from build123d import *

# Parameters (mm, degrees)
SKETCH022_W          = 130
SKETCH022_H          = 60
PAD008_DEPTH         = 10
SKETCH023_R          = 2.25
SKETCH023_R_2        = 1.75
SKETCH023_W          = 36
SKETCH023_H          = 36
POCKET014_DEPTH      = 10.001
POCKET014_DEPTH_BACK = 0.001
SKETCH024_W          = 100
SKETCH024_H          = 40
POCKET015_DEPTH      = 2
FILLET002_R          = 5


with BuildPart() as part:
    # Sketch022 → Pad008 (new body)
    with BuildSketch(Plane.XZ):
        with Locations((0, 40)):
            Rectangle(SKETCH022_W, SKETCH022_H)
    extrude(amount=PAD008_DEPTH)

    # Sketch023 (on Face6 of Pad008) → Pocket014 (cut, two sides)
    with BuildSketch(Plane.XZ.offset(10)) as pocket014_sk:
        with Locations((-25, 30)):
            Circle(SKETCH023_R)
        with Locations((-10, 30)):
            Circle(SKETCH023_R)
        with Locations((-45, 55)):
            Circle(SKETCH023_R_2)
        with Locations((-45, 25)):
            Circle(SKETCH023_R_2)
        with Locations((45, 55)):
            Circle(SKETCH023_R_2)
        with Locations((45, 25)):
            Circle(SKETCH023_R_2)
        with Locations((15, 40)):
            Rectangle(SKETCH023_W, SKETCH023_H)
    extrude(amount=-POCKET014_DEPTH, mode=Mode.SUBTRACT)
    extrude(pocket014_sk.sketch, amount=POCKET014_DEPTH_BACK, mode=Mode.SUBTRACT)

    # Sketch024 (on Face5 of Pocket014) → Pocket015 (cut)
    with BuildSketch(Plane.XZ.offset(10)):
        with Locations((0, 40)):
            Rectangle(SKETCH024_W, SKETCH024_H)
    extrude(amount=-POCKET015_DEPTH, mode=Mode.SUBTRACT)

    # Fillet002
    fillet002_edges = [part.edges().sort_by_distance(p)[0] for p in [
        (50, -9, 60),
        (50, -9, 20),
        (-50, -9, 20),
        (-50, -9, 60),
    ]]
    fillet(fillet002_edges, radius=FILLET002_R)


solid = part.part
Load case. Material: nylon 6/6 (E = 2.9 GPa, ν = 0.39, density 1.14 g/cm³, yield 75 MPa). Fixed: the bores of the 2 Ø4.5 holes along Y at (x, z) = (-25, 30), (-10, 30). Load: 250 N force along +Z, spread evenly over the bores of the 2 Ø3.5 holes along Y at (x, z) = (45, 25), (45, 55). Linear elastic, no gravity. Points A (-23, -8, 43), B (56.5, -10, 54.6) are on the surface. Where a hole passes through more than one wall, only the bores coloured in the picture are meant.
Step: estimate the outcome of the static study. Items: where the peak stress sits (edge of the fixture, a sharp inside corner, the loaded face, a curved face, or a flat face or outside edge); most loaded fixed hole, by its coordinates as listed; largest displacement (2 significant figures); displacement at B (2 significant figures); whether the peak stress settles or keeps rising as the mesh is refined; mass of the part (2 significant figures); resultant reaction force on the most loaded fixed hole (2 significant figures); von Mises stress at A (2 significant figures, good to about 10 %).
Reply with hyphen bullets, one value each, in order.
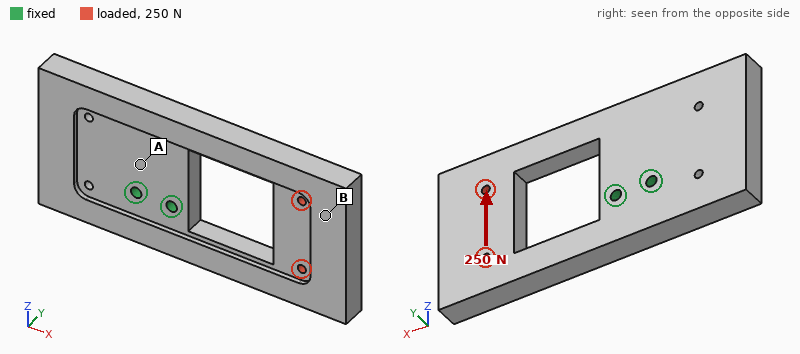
- edge of the fixture
- (-10, 30)
- 0.72 mm
- 0.67 mm
- keeps rising
- 67 g
- 1000 N
- 3.0 MPa
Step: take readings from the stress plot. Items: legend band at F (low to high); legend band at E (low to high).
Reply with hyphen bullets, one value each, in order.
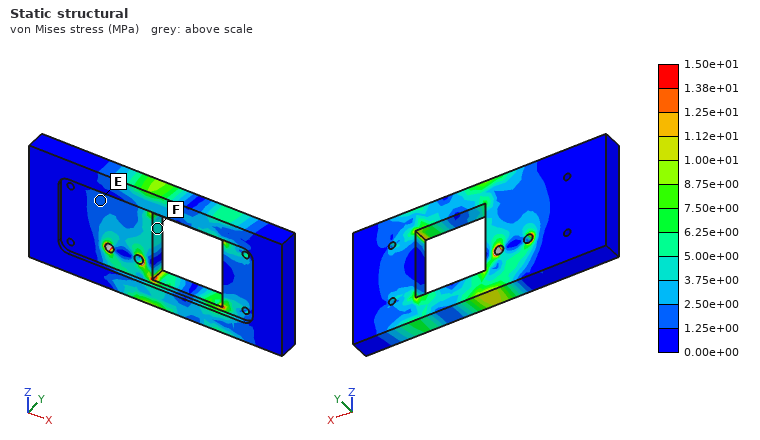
- 3.75e+00 to 5.00e+00 MPa
- 1.25e+00 to 2.50e+00 MPa
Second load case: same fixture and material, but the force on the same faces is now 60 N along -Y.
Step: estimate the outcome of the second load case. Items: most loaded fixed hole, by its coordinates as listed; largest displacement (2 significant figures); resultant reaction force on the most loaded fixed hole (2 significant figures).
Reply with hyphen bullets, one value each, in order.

- (-10, 30)
- 1.6 mm
- 190 N
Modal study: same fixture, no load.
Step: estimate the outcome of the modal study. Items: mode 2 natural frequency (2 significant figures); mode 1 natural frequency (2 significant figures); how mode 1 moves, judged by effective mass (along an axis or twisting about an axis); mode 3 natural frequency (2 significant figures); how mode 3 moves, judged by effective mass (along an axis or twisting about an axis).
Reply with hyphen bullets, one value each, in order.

- 590 Hz
- 230 Hz
- along Y
- 630 Hz
- along Z
